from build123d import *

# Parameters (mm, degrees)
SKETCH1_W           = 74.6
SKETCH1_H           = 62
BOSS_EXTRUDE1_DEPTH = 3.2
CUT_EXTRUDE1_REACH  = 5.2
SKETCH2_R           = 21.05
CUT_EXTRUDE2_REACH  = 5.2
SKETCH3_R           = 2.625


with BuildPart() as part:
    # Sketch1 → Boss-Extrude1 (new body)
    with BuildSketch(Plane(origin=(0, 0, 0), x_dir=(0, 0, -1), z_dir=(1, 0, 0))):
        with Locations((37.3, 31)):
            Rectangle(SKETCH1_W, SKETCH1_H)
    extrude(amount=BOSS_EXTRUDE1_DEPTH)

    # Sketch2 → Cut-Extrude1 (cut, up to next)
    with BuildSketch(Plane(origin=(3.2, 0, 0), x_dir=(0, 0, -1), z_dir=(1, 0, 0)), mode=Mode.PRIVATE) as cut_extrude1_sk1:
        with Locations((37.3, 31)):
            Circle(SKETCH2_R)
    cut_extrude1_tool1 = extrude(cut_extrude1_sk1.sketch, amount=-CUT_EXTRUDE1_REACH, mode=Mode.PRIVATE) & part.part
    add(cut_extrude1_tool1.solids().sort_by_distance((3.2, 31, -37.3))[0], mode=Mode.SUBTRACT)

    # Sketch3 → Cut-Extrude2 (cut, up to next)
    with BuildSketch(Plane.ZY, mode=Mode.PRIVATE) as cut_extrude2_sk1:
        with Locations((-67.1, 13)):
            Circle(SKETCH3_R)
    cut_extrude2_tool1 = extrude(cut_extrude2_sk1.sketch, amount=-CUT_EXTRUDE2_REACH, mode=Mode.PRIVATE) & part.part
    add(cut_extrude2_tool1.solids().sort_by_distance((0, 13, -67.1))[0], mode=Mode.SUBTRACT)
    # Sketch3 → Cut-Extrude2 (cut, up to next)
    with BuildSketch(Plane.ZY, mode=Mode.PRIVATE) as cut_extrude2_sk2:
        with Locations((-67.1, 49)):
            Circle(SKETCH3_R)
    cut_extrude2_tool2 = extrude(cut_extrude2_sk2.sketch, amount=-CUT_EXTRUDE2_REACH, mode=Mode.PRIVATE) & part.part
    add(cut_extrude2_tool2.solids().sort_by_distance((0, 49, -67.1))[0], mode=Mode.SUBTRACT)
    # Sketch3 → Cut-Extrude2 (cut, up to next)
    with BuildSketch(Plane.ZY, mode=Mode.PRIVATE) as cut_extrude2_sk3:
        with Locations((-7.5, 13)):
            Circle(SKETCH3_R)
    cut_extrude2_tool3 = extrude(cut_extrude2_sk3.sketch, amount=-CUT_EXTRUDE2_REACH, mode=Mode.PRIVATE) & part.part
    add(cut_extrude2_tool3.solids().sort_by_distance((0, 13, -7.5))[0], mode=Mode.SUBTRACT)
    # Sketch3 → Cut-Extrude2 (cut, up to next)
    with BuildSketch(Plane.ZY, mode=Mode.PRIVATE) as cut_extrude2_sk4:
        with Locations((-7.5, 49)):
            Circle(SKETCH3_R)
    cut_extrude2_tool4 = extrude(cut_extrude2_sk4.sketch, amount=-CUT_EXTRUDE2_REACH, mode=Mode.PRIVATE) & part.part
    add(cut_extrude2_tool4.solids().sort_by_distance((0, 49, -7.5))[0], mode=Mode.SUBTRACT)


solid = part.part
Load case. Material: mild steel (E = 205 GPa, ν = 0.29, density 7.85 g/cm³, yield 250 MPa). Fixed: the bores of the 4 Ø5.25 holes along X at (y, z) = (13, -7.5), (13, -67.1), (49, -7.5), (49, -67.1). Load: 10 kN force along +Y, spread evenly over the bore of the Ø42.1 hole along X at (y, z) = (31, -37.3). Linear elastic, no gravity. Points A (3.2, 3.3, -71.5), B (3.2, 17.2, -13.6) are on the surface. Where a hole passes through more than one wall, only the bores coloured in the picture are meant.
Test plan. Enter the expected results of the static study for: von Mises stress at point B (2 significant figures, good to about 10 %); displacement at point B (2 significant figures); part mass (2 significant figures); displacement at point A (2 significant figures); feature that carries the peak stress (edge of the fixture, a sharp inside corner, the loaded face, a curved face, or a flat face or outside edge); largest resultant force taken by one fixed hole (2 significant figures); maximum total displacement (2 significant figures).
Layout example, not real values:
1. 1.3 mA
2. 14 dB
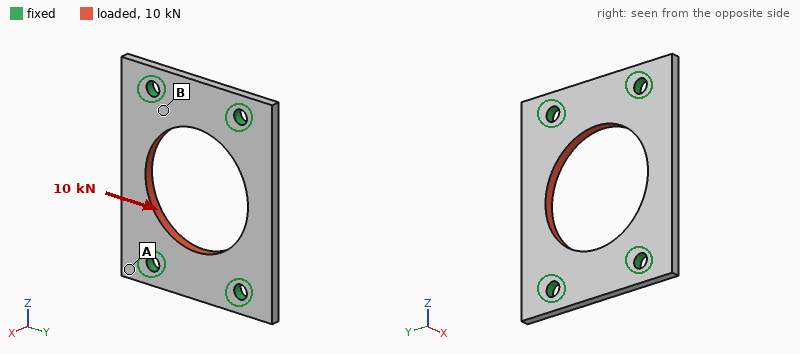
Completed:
1. 58 MPa
2. 3.4 µm
3. 79 g
4. 3.0 µm
5. edge of the fixture
6. 2.5 kN
7. 17 µm
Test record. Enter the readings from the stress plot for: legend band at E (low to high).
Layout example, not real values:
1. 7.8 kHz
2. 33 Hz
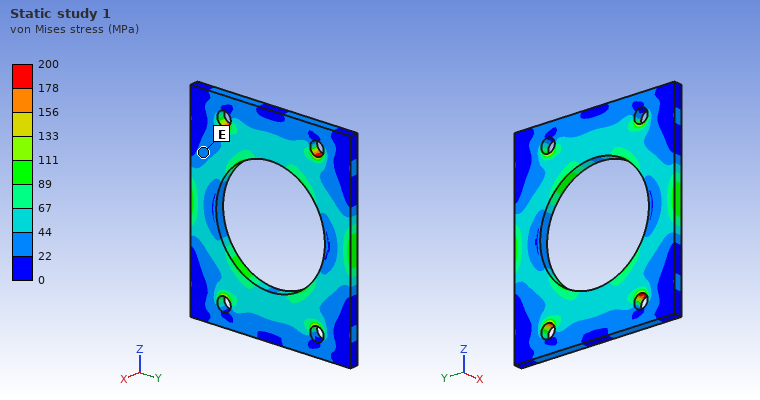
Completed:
1. 22 to 44 MPa
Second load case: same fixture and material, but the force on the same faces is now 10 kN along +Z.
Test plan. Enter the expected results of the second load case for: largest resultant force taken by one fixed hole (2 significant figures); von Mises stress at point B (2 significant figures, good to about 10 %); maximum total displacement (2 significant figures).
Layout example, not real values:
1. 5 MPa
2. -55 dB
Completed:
1. 2.5 kN
2. 43 MPa
3. 4.6 µm
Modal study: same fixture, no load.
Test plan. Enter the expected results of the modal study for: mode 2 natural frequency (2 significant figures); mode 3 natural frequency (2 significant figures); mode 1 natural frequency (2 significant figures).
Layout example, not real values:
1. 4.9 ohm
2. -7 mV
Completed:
1. 5300 Hz
2. 12 kHz
3. 5300 Hz
